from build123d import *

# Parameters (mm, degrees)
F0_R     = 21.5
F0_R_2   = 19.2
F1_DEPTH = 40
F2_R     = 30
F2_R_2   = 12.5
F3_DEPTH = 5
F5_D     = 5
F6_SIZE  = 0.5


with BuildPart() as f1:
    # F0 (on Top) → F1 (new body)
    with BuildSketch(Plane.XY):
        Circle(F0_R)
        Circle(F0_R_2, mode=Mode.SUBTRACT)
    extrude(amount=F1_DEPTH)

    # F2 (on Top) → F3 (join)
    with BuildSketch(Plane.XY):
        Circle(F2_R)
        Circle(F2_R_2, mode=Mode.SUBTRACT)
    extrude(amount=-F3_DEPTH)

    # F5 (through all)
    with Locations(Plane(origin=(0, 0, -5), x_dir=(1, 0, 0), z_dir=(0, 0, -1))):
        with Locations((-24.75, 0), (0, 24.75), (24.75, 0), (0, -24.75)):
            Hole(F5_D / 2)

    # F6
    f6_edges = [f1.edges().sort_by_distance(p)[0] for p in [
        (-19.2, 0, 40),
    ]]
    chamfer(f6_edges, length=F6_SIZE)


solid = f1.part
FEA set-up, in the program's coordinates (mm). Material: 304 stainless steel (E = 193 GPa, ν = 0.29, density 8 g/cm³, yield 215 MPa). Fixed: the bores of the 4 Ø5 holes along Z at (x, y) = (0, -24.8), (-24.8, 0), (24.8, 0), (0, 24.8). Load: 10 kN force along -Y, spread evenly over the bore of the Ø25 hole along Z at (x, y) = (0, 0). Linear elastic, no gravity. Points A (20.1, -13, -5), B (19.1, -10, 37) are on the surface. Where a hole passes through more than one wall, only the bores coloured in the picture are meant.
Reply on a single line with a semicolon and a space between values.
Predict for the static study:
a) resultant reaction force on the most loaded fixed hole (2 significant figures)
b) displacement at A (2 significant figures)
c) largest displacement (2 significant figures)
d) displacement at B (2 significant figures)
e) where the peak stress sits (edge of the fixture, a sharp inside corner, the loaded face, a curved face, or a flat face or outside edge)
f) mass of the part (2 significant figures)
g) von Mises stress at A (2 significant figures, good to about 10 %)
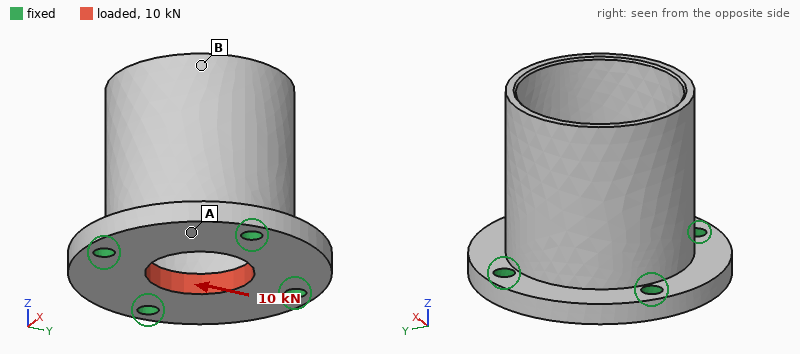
2.7 kN; 2.2 µm; 3.8 µm; 1.1 µm; edge of the fixture; 180 g; 15 MPa
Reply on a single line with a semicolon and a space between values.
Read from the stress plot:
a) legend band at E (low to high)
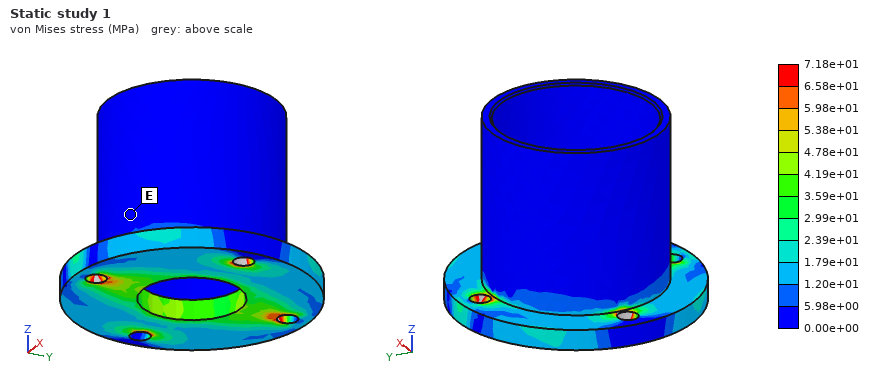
0.00e+00 to 5.98e+00 MPa
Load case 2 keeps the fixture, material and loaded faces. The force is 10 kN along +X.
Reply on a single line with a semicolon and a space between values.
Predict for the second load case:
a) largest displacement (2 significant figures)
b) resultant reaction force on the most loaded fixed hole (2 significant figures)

3.8 µm; 2.7 kN
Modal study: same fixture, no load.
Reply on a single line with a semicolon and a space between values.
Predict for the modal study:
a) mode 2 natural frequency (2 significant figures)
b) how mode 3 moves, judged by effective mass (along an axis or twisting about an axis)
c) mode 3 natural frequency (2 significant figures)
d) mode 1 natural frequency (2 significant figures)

6500 Hz; along X; 8700 Hz; 5100 Hz
